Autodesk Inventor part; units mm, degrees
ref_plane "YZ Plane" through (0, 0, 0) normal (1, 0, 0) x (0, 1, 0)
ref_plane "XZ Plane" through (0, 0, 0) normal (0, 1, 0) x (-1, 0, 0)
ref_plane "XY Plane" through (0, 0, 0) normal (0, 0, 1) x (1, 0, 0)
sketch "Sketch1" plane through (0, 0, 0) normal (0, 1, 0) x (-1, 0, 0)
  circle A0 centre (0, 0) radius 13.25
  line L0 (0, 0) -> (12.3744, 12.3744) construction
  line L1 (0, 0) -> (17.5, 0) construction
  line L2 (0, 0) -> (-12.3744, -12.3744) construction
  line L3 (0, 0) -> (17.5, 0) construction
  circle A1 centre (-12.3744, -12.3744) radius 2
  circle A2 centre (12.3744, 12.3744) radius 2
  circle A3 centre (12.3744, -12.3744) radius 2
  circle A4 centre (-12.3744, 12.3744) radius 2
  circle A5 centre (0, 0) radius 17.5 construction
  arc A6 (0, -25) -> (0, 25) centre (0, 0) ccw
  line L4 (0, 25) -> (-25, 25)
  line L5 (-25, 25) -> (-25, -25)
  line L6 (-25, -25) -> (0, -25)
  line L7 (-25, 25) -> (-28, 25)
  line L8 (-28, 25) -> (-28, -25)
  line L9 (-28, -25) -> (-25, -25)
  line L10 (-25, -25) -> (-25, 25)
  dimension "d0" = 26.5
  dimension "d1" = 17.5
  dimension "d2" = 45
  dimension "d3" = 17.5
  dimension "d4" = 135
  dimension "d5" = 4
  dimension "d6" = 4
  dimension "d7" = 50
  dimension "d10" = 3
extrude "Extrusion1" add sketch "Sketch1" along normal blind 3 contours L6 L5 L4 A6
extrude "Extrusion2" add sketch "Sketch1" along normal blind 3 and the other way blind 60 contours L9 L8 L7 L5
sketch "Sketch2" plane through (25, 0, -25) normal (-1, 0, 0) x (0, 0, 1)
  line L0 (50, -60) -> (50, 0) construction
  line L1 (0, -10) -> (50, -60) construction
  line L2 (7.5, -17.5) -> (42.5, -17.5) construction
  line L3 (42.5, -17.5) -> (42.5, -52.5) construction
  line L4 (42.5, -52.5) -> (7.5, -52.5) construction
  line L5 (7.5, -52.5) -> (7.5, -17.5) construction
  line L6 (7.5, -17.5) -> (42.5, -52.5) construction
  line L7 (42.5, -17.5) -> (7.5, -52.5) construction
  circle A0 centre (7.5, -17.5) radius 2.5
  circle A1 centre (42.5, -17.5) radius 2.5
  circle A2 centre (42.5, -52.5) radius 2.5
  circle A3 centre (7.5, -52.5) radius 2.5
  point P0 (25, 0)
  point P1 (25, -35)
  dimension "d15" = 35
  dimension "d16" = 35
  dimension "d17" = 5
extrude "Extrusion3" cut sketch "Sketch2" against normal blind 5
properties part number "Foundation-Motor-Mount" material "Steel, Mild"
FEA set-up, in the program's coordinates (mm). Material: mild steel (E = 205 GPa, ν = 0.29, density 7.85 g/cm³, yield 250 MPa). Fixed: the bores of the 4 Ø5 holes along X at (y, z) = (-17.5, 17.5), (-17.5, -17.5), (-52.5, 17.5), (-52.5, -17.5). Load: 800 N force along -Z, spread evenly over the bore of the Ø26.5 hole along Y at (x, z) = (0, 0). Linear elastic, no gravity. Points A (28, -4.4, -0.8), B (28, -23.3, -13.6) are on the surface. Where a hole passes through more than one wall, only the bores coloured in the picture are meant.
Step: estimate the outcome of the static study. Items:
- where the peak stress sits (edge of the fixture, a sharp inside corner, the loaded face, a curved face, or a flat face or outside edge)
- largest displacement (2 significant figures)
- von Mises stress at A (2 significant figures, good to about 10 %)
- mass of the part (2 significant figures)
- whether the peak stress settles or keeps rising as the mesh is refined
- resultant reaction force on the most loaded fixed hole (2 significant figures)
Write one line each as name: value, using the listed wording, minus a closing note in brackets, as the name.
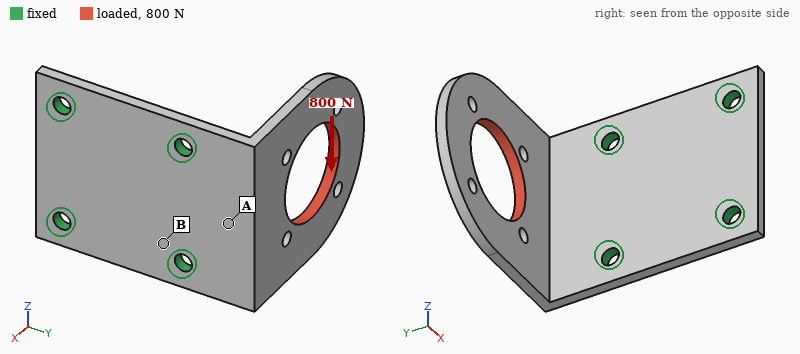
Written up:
where the peak stress sits: edge of the fixture
largest displacement: 0.18 mm
von Mises stress at A: 72 MPa
mass of the part: 110 g
whether the peak stress settles or keeps rising as the mesh is refined: keeps rising
resultant reaction force on the most loaded fixed hole: 790 N
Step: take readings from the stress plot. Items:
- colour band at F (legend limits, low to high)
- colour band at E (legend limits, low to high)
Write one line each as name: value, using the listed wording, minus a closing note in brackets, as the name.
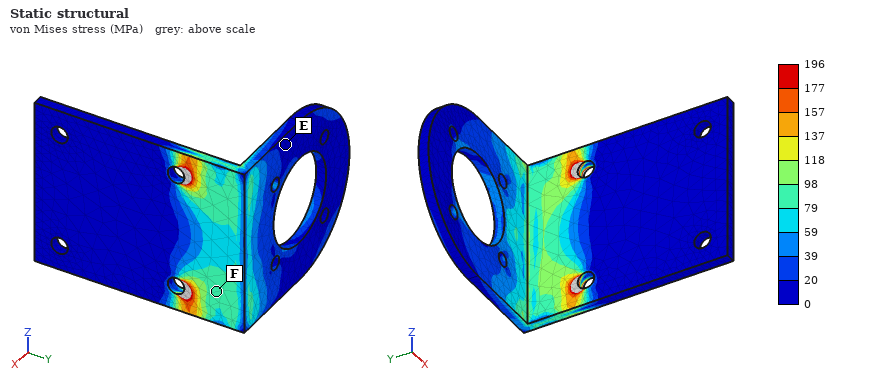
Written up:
colour band at F: 79 to 98 MPa
colour band at E: 0 to 20 MPa
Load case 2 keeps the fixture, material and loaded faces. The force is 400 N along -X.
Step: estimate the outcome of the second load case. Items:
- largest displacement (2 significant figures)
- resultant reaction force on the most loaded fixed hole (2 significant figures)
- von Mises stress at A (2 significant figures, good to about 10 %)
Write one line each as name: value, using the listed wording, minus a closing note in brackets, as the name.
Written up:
largest displacement: 0.16 mm
resultant reaction force on the most loaded fixed hole: 220 N
von Mises stress at A: 28 MPa
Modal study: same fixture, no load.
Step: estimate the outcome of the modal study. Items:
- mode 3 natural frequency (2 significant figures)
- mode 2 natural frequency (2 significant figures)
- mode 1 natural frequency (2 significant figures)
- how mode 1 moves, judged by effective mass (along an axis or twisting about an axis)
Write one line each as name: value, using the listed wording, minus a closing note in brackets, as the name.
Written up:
mode 3 natural frequency: 2700 Hz
mode 2 natural frequency: 1800 Hz
mode 1 natural frequency: 750 Hz
how mode 1 moves, judged by effective mass: along Y
